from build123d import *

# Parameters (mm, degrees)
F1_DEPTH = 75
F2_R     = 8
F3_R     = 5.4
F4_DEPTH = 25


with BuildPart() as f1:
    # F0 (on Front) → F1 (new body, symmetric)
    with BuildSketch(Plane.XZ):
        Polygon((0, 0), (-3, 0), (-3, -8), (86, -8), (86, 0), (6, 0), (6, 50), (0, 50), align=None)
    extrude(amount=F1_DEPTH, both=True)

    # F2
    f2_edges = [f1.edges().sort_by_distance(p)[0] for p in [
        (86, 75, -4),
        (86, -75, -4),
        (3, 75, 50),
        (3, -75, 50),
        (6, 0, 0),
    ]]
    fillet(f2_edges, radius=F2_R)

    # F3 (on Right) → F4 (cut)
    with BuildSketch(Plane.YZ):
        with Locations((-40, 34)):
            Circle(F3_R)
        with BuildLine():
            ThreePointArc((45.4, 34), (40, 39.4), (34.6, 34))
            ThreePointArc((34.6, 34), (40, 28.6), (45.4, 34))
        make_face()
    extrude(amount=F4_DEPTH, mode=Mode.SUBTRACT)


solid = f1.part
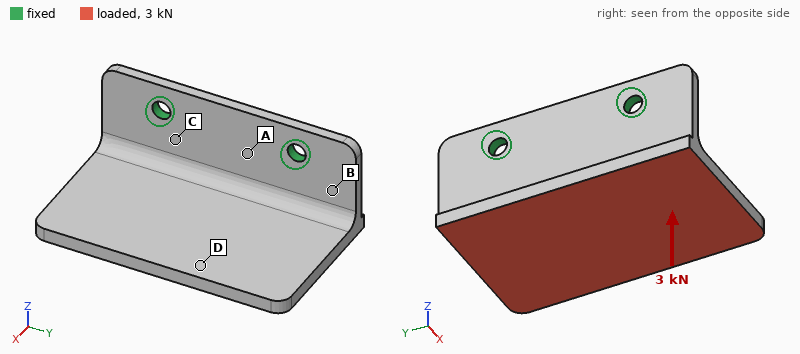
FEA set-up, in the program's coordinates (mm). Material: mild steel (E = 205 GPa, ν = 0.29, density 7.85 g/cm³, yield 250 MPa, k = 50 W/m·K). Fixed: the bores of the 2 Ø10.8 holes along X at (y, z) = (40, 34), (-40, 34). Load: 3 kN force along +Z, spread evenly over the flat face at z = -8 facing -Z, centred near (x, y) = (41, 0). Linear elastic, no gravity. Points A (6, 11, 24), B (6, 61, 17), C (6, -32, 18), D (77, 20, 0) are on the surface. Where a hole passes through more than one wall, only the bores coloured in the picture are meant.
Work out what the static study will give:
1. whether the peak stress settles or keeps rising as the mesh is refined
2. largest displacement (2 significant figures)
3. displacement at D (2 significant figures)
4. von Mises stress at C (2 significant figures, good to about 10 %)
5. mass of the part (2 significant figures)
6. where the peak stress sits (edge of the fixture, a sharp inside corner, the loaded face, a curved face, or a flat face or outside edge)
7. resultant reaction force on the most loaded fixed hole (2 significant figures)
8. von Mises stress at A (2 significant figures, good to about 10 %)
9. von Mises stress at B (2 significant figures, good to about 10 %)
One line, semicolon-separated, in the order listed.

keeps rising; 0.71 mm; 0.61 mm; 130 MPa; 1.2 kg; edge of the fixture; 1.5 kN; 86 MPa; 120 MPa
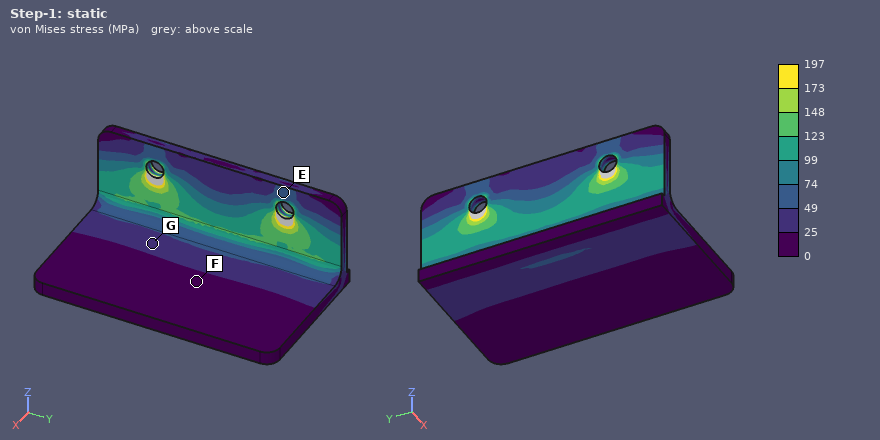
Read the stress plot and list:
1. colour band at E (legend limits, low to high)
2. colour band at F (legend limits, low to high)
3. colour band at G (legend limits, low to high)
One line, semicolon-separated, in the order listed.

49 to 74 MPa; 0 to 25 MPa; 25 to 49 MPa
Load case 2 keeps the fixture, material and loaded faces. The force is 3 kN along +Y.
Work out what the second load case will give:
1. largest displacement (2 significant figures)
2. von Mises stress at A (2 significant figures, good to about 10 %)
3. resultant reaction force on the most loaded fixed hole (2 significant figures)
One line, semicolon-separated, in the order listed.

92 µm; 23 MPa; 2.4 kN
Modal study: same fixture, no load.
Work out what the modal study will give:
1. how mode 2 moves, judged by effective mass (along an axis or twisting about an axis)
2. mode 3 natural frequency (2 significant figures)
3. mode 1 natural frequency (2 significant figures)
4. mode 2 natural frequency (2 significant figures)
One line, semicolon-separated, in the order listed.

along Y; 1500 Hz; 410 Hz; 910 Hz
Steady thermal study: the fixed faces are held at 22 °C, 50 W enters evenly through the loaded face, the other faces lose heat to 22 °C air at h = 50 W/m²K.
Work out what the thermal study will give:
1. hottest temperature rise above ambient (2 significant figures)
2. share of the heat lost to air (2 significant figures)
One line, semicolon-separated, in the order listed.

35 K; 62 %
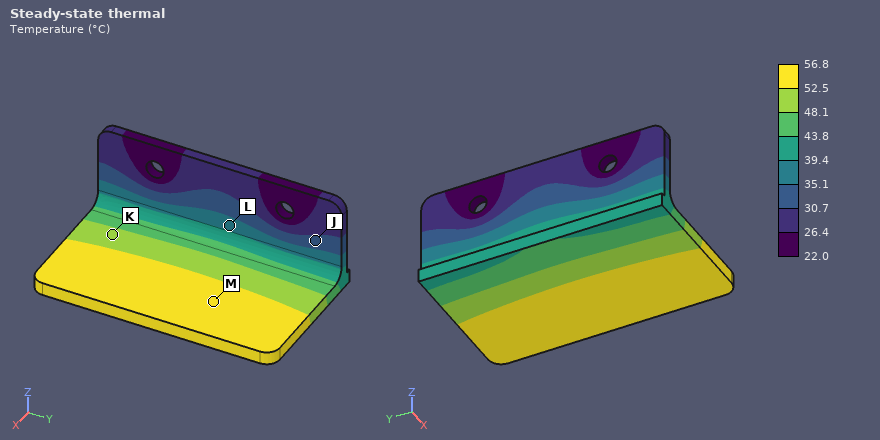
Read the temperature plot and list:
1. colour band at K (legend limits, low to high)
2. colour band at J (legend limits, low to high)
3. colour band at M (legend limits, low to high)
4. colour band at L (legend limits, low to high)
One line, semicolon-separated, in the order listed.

48.1 to 52.5 °C; 30.7 to 35.1 °C; 52.5 to 56.8 °C; 35.1 to 39.4 °C
